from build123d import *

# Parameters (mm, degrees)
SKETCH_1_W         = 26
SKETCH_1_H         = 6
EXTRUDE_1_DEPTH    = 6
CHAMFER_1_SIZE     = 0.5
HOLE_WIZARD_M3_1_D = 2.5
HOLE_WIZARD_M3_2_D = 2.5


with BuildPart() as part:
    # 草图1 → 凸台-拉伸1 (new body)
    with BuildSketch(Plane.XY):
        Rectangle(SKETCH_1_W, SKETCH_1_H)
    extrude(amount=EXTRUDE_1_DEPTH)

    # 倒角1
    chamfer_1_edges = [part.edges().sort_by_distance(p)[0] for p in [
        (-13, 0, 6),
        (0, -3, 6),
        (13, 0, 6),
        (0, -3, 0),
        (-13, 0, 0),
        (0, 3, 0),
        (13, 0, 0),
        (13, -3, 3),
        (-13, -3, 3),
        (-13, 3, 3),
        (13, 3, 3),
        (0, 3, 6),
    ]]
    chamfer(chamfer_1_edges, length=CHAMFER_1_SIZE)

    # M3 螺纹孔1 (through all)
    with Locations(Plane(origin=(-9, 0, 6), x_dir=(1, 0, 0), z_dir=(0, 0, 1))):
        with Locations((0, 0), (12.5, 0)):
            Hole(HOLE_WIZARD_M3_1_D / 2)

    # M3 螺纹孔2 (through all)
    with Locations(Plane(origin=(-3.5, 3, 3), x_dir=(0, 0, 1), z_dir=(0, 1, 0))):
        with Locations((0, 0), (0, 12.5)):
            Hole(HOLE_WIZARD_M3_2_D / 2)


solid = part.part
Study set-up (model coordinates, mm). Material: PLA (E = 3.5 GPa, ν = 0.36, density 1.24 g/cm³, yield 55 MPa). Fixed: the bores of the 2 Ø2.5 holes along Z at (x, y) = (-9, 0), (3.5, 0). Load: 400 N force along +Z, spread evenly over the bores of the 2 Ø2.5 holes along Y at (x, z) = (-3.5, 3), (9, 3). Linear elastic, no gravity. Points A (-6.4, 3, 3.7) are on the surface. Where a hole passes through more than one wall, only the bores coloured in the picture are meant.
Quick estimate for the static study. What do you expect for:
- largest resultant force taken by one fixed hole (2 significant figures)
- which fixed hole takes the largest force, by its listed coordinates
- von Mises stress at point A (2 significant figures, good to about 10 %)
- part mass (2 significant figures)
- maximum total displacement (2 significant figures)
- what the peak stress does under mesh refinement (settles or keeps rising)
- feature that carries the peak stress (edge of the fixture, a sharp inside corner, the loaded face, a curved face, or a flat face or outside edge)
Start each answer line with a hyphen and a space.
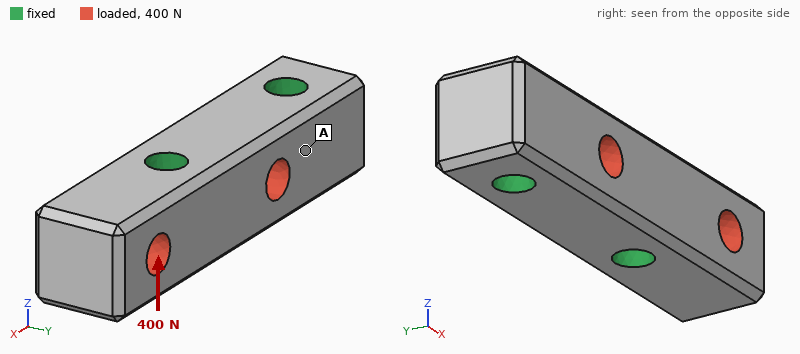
- 290 N
- (3.5, 0)
- 6.5 MPa
- 0.99 g
- 91 µm
- keeps rising
- edge of the fixture
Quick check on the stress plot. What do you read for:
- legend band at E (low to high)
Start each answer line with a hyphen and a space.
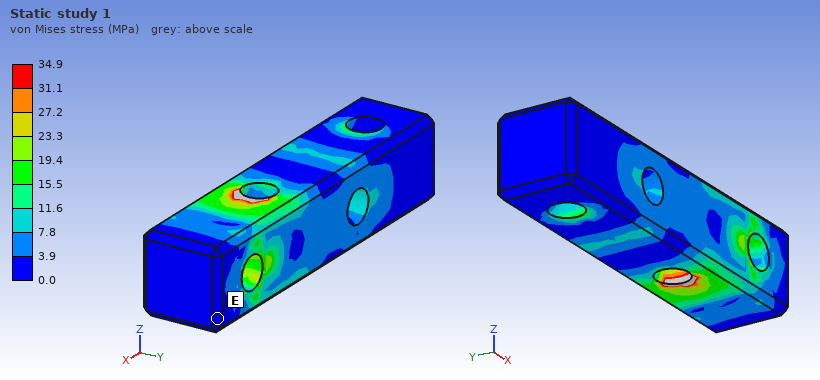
- 0.0 to 3.9 MPa
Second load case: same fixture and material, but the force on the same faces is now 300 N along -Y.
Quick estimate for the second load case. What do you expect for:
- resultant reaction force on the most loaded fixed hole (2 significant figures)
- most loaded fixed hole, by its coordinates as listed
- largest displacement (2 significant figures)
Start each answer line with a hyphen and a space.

- 230 N
- (3.5, 0)
- 88 µm
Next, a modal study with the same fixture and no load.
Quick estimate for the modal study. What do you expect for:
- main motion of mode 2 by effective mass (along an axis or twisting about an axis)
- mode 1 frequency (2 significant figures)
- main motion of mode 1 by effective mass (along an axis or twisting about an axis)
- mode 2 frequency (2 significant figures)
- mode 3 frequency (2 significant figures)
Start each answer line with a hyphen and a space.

- along Z
- 13 kHz
- along Y
- 15 kHz
- 25 kHz
